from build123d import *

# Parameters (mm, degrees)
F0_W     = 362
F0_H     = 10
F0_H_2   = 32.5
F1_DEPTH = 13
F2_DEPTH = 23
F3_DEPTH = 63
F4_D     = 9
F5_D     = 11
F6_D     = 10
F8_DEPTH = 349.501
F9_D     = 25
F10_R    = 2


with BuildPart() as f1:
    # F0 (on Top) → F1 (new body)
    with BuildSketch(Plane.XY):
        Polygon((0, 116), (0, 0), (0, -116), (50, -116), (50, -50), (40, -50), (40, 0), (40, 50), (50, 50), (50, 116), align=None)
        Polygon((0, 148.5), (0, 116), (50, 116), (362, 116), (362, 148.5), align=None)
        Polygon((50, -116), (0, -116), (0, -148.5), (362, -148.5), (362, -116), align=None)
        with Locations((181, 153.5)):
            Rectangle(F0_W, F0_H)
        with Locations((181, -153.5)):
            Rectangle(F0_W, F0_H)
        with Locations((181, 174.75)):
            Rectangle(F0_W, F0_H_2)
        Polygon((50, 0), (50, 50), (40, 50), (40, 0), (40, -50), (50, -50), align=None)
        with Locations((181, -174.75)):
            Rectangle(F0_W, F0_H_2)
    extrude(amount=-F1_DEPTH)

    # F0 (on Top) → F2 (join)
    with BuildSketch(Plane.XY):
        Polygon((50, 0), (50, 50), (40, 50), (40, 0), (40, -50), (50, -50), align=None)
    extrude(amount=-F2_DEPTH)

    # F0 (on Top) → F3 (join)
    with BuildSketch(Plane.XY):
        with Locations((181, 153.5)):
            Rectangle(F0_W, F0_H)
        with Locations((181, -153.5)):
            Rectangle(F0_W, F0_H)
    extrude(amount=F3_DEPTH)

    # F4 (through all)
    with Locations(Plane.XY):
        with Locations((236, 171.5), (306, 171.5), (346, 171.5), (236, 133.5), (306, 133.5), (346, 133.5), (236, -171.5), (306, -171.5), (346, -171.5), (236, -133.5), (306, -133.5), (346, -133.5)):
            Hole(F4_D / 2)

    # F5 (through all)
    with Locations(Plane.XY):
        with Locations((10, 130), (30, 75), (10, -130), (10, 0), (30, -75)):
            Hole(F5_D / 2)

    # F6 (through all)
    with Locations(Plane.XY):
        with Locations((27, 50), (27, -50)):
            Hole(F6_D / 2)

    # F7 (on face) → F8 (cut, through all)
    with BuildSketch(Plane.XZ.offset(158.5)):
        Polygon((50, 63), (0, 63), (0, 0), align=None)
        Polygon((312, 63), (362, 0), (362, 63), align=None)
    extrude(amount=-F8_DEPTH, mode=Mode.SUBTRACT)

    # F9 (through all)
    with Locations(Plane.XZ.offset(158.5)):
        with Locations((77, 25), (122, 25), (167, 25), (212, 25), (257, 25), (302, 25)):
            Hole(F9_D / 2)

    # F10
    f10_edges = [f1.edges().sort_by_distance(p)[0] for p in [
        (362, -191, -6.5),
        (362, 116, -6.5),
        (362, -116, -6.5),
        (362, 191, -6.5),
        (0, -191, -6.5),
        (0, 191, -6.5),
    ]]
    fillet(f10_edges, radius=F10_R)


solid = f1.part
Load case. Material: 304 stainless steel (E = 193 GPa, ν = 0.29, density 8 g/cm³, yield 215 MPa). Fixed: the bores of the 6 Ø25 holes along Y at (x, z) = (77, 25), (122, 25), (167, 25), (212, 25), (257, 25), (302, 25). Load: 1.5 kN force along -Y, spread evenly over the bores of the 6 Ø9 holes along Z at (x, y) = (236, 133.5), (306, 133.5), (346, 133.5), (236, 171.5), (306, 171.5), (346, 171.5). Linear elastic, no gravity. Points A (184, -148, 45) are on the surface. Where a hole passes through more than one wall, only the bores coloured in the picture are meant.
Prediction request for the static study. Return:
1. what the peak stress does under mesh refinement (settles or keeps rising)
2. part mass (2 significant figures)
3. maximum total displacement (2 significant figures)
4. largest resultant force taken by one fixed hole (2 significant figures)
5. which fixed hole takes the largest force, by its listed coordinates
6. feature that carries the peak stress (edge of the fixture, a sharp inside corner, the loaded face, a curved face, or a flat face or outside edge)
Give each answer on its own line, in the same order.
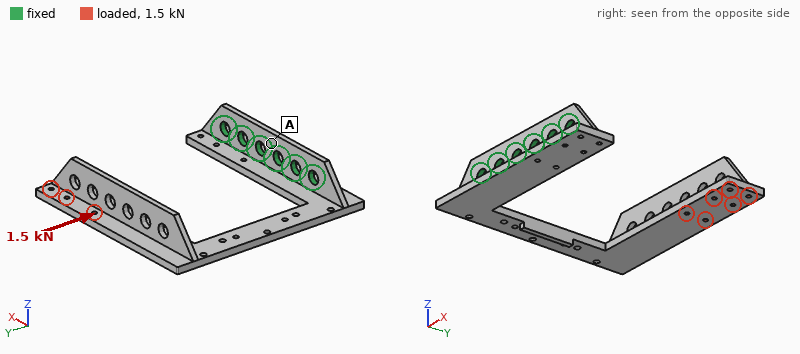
keeps rising
9.5 kg
2.0 mm
1.5 kN
(77, 25)
a sharp inside corner
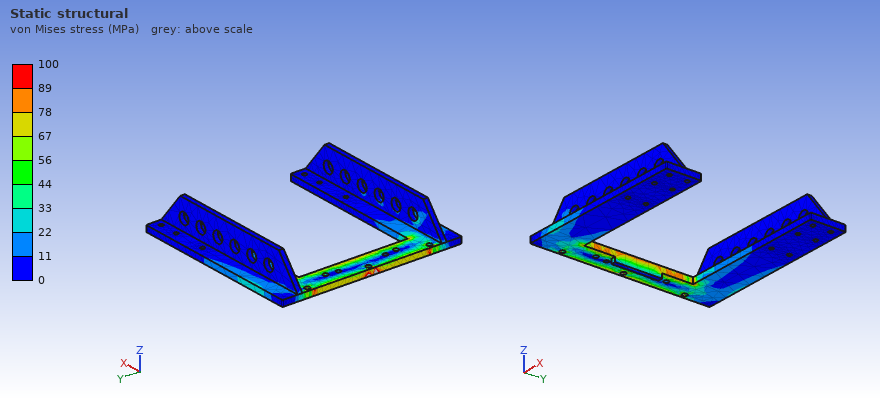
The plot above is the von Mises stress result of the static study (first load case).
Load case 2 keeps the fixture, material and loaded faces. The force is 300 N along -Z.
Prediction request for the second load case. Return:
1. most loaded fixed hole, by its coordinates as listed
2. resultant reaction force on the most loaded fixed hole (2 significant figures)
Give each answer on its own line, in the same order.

(77, 25)
850 N
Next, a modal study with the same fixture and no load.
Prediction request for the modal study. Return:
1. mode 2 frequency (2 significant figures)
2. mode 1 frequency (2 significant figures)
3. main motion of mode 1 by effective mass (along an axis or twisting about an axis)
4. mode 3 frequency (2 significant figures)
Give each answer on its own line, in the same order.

73 Hz
26 Hz
along Z
91 Hz
